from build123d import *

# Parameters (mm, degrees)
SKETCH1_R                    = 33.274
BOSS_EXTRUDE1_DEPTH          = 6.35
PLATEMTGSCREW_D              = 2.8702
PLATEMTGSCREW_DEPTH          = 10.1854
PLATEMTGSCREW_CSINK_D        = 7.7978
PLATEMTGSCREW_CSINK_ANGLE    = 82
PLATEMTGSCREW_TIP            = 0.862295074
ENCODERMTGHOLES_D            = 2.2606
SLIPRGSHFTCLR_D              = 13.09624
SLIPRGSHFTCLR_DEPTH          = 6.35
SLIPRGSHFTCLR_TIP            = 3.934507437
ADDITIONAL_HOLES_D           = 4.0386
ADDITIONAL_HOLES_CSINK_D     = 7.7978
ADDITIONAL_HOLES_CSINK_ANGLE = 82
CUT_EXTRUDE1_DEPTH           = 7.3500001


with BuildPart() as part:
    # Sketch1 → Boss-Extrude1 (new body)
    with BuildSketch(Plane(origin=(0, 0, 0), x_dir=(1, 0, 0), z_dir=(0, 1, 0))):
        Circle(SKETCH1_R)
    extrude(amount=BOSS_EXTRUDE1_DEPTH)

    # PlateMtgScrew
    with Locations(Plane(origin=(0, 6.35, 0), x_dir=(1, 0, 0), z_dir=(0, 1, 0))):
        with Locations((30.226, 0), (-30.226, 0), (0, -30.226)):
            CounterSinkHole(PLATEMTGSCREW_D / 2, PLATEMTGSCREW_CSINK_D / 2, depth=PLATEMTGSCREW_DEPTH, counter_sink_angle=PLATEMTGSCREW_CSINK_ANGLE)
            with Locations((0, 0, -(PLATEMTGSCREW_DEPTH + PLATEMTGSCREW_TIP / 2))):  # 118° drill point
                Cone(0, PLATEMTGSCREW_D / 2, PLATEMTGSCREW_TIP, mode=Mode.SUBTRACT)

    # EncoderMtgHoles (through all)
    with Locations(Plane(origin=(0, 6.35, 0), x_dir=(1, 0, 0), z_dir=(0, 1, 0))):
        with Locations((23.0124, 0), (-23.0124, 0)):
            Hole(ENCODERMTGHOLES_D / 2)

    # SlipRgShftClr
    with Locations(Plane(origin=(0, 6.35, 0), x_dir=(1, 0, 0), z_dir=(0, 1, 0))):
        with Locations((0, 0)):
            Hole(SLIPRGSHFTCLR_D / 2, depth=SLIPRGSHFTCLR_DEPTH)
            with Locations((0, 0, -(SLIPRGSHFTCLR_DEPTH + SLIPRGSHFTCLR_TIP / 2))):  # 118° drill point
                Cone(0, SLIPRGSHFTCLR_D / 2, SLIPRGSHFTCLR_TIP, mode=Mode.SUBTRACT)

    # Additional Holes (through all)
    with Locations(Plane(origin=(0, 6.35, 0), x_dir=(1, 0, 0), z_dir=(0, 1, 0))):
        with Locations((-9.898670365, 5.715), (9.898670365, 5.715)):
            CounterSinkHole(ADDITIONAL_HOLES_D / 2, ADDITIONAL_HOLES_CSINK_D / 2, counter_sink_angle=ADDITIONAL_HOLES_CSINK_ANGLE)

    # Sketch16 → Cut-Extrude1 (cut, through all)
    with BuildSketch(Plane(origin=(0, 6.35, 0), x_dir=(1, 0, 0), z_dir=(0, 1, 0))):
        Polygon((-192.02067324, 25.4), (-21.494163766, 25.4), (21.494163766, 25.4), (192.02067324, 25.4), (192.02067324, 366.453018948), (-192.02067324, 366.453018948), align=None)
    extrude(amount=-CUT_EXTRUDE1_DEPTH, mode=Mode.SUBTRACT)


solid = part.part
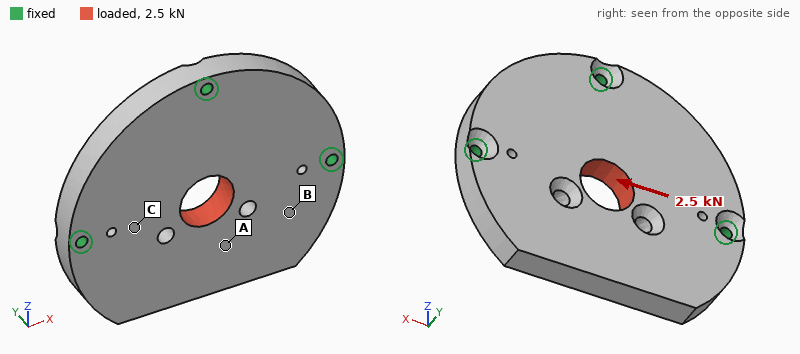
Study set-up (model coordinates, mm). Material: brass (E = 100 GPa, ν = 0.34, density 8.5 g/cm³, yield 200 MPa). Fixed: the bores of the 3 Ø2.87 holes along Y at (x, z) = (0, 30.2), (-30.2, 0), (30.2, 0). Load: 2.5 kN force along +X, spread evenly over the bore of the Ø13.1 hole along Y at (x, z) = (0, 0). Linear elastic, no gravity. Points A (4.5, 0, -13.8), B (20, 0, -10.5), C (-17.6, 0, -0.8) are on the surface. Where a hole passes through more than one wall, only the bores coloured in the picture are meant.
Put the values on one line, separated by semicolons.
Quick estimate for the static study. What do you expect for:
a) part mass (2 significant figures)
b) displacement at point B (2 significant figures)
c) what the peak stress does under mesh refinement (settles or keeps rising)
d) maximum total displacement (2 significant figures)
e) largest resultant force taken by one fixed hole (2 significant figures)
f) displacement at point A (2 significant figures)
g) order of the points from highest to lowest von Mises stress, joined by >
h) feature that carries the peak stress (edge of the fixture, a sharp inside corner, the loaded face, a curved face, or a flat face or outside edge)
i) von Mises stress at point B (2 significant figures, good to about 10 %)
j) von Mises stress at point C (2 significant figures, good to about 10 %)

160 g; 2.9 µm; keeps rising; 4.6 µm; 1.0 kN; 3.5 µm; C > B > A; edge of the fixture; 7.4 MPa; 12 MPa
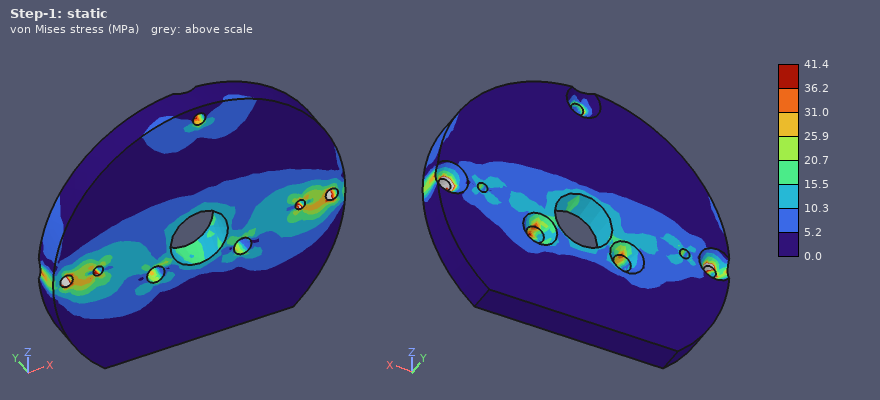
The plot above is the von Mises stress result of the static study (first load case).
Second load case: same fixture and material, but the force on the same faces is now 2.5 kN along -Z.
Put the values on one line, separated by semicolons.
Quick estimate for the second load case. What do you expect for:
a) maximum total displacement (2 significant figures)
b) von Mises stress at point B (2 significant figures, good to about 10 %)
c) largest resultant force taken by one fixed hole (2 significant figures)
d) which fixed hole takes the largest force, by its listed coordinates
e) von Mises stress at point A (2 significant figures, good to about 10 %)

7.0 µm; 6.2 MPa; 1.0 kN; (0, 30.2); 8.1 MPa
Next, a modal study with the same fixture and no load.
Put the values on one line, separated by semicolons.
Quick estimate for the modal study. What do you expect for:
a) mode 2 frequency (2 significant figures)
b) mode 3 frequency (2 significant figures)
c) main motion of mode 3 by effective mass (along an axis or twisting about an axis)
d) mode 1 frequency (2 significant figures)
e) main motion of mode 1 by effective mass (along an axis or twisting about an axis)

6100 Hz; 6600 Hz; along Y; 2500 Hz; along Y
